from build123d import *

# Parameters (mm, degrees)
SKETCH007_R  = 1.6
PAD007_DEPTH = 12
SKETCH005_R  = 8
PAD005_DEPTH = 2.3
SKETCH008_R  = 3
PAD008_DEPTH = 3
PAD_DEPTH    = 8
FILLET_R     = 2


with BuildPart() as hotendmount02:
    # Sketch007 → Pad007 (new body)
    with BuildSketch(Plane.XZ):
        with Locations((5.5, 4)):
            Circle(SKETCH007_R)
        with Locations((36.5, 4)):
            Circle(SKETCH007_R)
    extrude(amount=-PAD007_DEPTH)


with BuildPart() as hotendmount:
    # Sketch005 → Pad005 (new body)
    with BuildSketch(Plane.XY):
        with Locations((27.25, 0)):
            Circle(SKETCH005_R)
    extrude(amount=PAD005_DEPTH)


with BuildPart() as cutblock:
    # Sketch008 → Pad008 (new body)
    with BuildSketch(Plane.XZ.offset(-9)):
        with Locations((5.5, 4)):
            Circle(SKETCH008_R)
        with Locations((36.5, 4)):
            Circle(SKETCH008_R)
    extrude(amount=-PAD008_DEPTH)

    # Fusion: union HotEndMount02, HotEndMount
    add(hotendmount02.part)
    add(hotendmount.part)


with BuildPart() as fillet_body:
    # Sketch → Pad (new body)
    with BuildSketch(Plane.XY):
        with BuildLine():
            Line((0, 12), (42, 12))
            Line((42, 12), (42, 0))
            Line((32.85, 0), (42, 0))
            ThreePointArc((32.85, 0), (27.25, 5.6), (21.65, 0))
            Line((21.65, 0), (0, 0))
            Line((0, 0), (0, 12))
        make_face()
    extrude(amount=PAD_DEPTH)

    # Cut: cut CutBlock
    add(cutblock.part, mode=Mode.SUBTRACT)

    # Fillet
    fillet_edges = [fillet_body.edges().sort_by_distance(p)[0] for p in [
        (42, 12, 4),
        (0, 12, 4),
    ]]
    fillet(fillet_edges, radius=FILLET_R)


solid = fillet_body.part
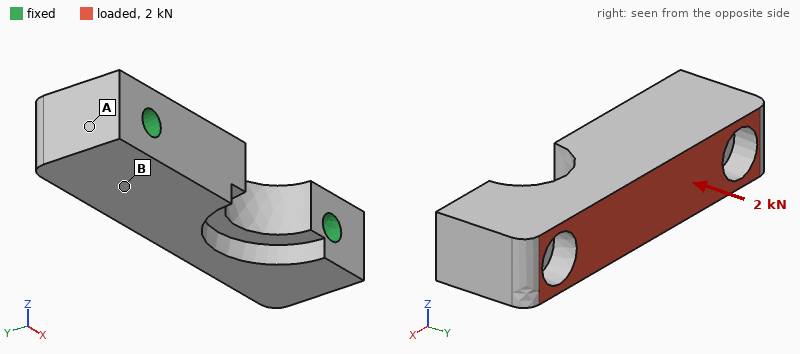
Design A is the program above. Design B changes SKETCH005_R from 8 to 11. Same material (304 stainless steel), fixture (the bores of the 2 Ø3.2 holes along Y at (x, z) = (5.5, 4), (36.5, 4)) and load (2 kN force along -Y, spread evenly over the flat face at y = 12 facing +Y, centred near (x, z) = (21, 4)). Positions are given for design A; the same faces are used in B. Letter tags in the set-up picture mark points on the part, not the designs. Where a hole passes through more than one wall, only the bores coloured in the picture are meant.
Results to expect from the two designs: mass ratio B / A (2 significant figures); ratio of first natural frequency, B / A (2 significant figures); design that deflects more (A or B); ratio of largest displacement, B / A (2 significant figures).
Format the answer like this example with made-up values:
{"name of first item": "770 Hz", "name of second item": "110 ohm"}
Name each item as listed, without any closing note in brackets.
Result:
{"mass ratio B / A": "0.94", "ratio of first natural frequency, B / A": "0.97", "design that deflects more": "B", "ratio of largest displacement, B / A": "1.5"}
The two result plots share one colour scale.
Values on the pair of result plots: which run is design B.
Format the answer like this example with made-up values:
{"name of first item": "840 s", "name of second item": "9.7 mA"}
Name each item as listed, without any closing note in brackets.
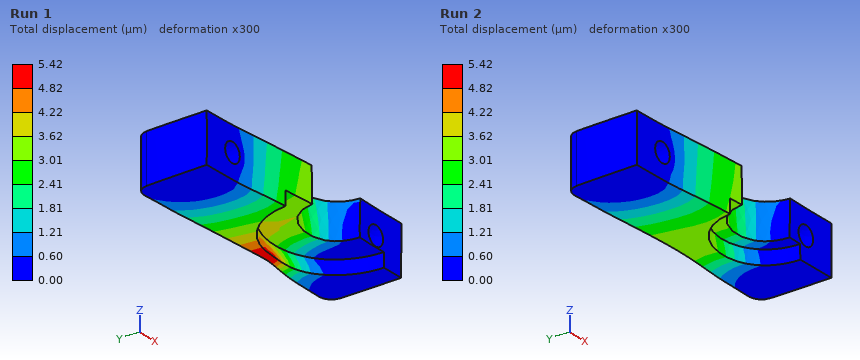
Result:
{"which run is design B": "Run 1"}
